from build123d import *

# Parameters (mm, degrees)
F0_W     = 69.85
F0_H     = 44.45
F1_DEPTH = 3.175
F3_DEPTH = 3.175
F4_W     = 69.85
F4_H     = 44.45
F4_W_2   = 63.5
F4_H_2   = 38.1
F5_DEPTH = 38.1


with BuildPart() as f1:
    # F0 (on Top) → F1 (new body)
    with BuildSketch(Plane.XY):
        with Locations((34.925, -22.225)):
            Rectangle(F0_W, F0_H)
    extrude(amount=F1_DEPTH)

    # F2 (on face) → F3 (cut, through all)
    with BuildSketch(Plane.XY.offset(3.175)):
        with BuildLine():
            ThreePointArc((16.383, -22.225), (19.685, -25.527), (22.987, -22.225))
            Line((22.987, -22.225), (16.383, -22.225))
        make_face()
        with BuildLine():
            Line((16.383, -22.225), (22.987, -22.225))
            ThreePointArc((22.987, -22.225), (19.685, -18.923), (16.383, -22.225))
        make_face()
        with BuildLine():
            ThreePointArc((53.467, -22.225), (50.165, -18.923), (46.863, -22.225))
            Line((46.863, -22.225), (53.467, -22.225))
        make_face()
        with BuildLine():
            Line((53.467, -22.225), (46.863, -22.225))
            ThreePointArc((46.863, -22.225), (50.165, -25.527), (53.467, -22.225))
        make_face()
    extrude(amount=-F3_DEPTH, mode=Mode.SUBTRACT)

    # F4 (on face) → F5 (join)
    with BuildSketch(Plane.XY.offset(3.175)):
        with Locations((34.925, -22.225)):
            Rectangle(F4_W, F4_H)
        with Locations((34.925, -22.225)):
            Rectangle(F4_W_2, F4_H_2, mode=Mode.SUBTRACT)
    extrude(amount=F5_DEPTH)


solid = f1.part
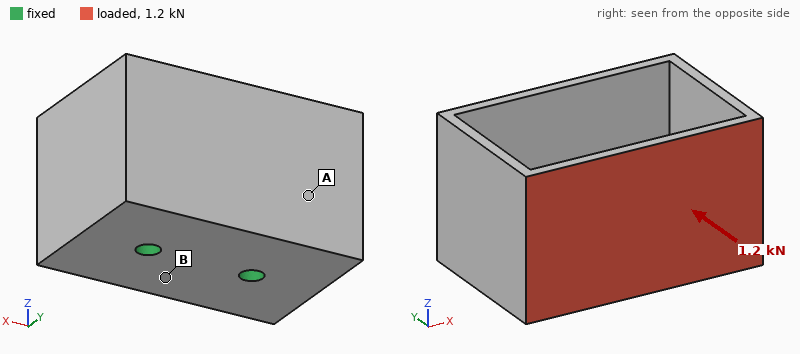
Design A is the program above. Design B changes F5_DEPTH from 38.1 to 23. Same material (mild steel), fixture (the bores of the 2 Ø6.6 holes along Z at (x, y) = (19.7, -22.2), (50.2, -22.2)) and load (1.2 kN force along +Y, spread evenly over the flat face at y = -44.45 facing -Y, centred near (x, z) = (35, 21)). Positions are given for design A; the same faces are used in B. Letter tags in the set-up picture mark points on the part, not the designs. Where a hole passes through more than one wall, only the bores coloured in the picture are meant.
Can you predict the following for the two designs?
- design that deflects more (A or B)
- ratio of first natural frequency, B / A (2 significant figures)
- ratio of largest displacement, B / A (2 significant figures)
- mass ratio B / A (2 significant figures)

A
1.6
0.58
0.71
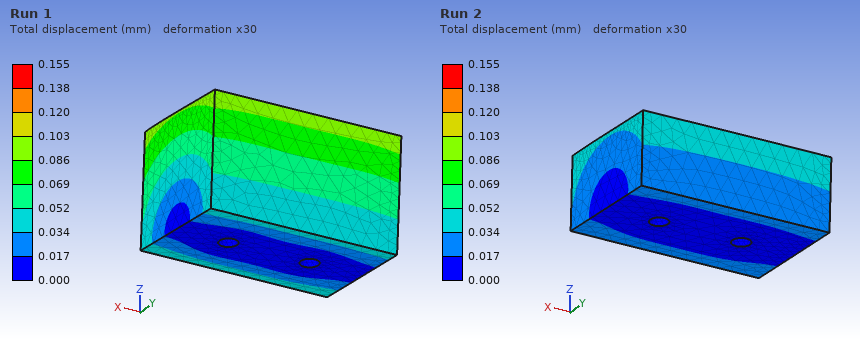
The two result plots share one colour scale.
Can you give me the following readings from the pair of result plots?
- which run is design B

Run 2
